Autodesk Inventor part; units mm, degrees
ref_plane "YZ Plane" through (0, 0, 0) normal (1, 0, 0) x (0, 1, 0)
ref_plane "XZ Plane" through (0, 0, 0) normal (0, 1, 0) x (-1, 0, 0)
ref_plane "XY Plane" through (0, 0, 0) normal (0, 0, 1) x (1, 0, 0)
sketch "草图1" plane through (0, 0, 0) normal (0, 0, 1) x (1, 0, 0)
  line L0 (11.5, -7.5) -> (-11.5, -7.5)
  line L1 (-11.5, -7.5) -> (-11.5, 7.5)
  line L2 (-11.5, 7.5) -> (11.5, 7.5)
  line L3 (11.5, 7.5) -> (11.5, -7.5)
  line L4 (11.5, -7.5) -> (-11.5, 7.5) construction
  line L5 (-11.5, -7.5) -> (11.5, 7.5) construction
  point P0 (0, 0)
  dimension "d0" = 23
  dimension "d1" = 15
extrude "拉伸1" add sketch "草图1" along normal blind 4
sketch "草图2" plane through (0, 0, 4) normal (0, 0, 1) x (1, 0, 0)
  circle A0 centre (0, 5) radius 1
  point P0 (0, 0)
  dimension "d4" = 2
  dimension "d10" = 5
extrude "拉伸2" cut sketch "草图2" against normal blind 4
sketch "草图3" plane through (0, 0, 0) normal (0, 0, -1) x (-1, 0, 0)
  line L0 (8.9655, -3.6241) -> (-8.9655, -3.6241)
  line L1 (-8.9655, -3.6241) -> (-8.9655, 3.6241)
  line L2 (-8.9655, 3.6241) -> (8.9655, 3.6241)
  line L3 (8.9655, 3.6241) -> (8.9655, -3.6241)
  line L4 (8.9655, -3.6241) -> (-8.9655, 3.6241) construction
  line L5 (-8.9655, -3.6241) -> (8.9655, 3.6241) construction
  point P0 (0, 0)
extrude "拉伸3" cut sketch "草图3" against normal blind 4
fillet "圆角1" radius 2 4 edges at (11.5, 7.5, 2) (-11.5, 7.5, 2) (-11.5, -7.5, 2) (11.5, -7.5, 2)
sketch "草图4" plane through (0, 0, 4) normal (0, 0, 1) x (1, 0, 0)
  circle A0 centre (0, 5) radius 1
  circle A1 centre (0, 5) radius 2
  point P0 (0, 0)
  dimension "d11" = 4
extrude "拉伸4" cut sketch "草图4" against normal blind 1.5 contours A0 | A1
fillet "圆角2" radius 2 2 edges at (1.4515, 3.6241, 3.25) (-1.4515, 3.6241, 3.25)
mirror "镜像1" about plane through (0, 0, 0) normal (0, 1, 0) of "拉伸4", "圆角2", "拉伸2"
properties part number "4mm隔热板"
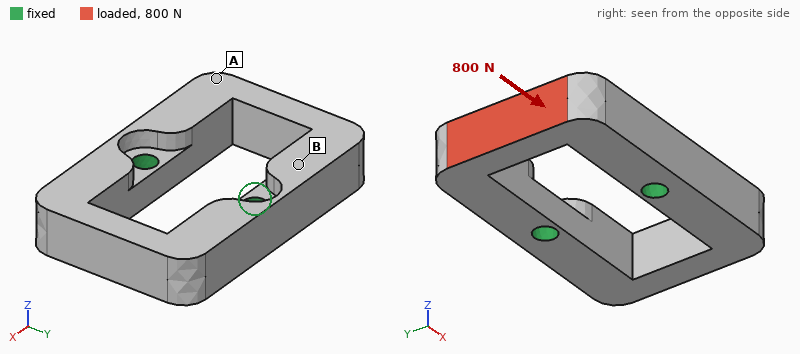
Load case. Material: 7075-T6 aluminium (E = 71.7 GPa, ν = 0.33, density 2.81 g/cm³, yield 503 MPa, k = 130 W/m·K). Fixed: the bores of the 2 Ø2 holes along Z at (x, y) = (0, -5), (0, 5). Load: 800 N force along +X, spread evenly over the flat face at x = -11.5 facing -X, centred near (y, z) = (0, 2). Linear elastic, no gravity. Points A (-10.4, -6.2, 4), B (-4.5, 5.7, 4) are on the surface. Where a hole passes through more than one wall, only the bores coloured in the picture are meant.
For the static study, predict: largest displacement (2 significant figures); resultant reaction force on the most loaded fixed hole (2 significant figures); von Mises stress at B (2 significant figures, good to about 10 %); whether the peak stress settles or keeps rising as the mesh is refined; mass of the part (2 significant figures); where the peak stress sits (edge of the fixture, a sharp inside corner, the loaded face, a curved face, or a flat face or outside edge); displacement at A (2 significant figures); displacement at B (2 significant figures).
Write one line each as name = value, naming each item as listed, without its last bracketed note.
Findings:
largest displacement = 22 µm
resultant reaction force on the most loaded fixed hole = 410 N
von Mises stress at B = 34 MPa
whether the peak stress settles or keeps rising as the mesh is refined = keeps rising
mass of the part = 2.2 g
where the peak stress sits = edge of the fixture
displacement at A = 12 µm
displacement at B = 7.2 µm
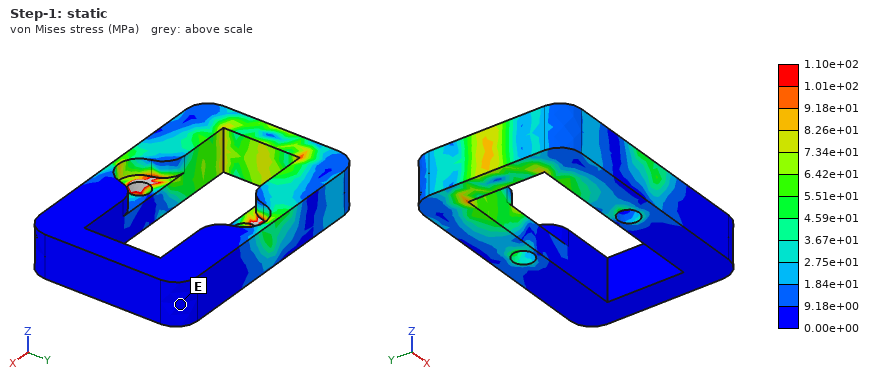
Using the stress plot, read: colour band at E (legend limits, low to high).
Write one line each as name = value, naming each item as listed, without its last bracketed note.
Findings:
colour band at E = 0.00e+00 to 9.18e+00 MPa
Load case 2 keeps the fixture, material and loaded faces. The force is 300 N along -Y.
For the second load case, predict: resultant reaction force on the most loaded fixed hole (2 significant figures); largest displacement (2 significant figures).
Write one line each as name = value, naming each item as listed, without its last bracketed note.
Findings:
resultant reaction force on the most loaded fixed hole = 220 N
largest displacement = 31 µm
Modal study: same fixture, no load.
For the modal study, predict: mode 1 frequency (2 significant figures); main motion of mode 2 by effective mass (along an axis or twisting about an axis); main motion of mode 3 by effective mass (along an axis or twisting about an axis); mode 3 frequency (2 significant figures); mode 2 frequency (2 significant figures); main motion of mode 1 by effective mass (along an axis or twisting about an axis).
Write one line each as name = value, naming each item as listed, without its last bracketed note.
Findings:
mode 1 frequency = 13 kHz
main motion of mode 2 by effective mass = along Z
main motion of mode 3 by effective mass = twisting about Z
mode 3 frequency = 20 kHz
mode 2 frequency = 15 kHz
main motion of mode 1 by effective mass = twisting about Y
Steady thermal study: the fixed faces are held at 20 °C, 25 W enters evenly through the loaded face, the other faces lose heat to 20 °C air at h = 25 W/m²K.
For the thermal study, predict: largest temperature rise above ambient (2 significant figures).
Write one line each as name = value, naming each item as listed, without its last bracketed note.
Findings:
largest temperature rise above ambient = 86 K
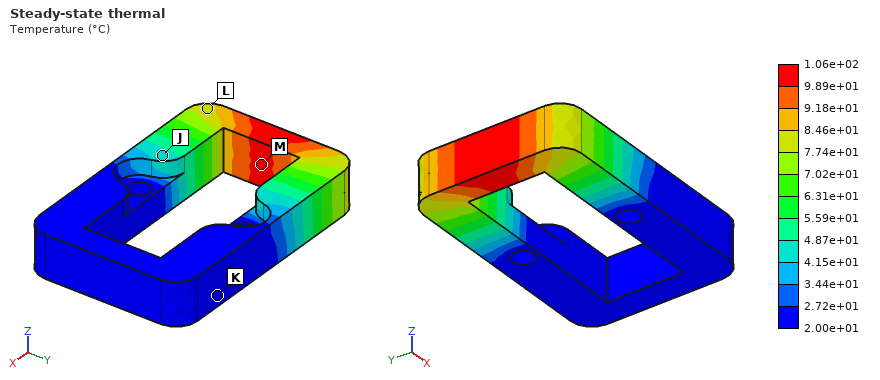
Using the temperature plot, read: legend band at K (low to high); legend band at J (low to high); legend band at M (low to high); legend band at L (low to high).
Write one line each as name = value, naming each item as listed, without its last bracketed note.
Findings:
legend band at K = 2.00e+01 to 2.72e+01 °C
legend band at J = 4.15e+01 to 4.87e+01 °C
legend band at M = 9.89e+01 to 1.06e+02 °C
legend band at L = 7.74e+01 to 8.46e+01 °C
